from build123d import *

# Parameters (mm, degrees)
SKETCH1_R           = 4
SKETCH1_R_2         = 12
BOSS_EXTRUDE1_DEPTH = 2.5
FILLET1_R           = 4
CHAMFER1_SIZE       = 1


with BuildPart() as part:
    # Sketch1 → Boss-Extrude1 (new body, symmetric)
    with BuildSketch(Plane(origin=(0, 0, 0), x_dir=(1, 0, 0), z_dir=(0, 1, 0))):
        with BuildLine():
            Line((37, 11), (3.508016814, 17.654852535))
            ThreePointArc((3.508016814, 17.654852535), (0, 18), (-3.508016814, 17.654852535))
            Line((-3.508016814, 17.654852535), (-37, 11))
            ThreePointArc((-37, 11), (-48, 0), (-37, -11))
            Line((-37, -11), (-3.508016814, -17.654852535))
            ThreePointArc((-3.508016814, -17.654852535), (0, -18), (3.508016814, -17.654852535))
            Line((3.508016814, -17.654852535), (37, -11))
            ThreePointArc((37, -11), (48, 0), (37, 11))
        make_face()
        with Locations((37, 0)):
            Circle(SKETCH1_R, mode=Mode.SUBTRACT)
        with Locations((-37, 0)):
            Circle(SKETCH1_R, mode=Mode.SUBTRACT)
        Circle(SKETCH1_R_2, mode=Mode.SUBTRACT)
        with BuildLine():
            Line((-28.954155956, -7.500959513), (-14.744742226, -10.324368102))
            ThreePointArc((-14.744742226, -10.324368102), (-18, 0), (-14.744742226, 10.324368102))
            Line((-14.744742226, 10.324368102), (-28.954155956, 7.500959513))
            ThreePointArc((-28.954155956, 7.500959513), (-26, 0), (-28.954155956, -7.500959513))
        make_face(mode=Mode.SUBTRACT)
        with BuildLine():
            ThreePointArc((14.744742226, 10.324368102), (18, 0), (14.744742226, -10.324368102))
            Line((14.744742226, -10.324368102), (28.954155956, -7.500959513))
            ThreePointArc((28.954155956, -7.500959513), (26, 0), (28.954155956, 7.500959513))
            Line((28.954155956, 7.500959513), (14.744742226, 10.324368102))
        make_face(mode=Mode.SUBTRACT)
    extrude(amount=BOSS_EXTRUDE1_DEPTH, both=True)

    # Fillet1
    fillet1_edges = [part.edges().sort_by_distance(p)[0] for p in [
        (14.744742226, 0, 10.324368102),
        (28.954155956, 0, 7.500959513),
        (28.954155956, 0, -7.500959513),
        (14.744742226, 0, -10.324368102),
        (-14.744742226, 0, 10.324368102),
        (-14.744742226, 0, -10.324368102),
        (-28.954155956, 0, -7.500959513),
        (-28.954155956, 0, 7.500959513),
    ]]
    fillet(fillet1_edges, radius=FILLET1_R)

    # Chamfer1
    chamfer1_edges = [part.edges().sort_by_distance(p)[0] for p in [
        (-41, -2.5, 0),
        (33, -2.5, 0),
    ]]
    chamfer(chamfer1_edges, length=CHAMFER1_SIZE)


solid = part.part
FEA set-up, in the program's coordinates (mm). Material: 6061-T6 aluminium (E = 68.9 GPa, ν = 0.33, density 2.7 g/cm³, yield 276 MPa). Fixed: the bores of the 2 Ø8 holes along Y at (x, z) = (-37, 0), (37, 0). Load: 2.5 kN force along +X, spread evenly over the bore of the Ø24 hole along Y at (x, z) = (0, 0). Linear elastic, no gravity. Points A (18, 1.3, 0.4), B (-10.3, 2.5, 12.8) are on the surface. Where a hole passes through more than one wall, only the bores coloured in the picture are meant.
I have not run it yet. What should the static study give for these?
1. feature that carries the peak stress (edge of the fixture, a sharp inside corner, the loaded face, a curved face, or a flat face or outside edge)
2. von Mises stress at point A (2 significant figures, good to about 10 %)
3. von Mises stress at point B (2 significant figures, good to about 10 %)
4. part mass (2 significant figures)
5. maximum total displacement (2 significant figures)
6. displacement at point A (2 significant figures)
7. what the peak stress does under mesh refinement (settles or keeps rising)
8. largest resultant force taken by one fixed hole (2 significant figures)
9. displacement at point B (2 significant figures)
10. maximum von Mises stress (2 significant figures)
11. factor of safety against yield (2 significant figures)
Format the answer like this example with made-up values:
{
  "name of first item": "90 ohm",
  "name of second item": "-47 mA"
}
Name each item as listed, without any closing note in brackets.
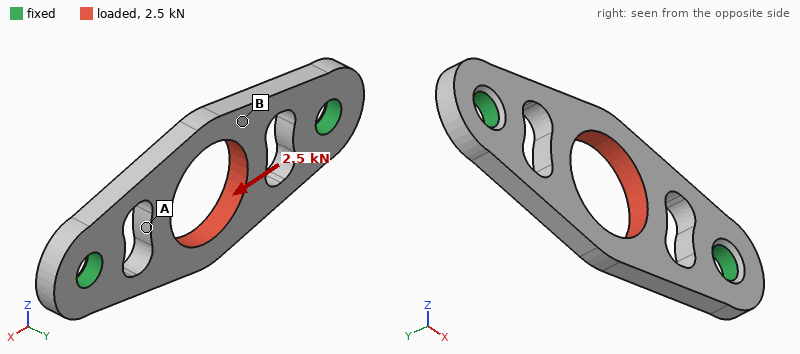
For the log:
{
  "feature that carries the peak stress": "a curved face",
  "von Mises stress at point A": "22 MPa",
  "von Mises stress at point B": "11 MPa",
  "part mass": "23 g",
  "maximum total displacement": "14 µm",
  "displacement at point A": "14 µm",
  "what the peak stress does under mesh refinement": "settles",
  "largest resultant force taken by one fixed hole": "1.3 kN",
  "displacement at point B": "9.3 µm",
  "maximum von Mises stress": "67 MPa",
  "factor of safety against yield": "4.1"
}
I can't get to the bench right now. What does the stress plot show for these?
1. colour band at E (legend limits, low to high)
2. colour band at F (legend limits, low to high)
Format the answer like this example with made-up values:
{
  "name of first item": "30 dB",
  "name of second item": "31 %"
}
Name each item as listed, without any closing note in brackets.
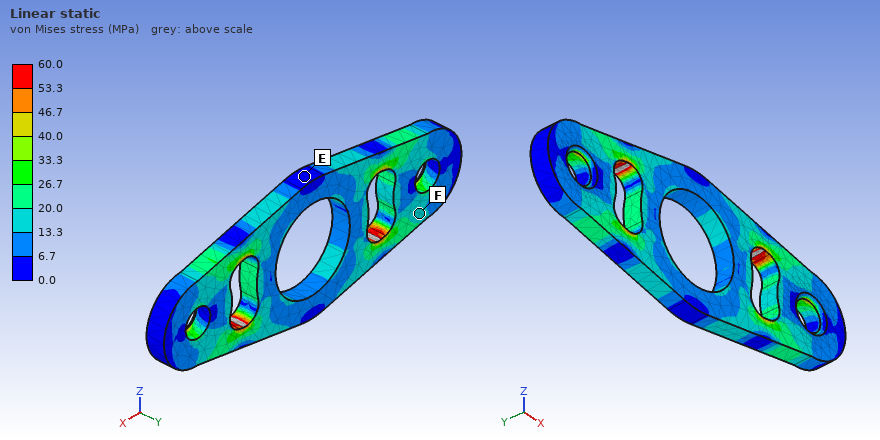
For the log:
{
  "colour band at E": "0.0 to 6.7 MPa",
  "colour band at F": "13.3 to 20.0 MPa"
}
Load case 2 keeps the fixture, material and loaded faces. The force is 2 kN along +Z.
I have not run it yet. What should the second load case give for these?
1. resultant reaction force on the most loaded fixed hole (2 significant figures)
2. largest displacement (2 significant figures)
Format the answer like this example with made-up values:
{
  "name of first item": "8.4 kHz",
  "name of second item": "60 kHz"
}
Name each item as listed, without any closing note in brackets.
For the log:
{
  "resultant reaction force on the most loaded fixed hole": "1.0 kN",
  "largest displacement": "44 µm"
}
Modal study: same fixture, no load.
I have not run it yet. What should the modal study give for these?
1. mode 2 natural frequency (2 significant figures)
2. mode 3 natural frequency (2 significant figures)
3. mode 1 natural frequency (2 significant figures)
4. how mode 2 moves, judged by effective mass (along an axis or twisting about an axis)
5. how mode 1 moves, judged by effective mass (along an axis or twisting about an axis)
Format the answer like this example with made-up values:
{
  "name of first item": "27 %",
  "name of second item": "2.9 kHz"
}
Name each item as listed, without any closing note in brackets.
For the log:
{
  "mode 2 natural frequency": "5200 Hz",
  "mode 3 natural frequency": "10 kHz",
  "mode 1 natural frequency": "4300 Hz",
  "how mode 2 moves, judged by effective mass": "twisting about X",
  "how mode 1 moves, judged by effective mass": "along Y"
}
